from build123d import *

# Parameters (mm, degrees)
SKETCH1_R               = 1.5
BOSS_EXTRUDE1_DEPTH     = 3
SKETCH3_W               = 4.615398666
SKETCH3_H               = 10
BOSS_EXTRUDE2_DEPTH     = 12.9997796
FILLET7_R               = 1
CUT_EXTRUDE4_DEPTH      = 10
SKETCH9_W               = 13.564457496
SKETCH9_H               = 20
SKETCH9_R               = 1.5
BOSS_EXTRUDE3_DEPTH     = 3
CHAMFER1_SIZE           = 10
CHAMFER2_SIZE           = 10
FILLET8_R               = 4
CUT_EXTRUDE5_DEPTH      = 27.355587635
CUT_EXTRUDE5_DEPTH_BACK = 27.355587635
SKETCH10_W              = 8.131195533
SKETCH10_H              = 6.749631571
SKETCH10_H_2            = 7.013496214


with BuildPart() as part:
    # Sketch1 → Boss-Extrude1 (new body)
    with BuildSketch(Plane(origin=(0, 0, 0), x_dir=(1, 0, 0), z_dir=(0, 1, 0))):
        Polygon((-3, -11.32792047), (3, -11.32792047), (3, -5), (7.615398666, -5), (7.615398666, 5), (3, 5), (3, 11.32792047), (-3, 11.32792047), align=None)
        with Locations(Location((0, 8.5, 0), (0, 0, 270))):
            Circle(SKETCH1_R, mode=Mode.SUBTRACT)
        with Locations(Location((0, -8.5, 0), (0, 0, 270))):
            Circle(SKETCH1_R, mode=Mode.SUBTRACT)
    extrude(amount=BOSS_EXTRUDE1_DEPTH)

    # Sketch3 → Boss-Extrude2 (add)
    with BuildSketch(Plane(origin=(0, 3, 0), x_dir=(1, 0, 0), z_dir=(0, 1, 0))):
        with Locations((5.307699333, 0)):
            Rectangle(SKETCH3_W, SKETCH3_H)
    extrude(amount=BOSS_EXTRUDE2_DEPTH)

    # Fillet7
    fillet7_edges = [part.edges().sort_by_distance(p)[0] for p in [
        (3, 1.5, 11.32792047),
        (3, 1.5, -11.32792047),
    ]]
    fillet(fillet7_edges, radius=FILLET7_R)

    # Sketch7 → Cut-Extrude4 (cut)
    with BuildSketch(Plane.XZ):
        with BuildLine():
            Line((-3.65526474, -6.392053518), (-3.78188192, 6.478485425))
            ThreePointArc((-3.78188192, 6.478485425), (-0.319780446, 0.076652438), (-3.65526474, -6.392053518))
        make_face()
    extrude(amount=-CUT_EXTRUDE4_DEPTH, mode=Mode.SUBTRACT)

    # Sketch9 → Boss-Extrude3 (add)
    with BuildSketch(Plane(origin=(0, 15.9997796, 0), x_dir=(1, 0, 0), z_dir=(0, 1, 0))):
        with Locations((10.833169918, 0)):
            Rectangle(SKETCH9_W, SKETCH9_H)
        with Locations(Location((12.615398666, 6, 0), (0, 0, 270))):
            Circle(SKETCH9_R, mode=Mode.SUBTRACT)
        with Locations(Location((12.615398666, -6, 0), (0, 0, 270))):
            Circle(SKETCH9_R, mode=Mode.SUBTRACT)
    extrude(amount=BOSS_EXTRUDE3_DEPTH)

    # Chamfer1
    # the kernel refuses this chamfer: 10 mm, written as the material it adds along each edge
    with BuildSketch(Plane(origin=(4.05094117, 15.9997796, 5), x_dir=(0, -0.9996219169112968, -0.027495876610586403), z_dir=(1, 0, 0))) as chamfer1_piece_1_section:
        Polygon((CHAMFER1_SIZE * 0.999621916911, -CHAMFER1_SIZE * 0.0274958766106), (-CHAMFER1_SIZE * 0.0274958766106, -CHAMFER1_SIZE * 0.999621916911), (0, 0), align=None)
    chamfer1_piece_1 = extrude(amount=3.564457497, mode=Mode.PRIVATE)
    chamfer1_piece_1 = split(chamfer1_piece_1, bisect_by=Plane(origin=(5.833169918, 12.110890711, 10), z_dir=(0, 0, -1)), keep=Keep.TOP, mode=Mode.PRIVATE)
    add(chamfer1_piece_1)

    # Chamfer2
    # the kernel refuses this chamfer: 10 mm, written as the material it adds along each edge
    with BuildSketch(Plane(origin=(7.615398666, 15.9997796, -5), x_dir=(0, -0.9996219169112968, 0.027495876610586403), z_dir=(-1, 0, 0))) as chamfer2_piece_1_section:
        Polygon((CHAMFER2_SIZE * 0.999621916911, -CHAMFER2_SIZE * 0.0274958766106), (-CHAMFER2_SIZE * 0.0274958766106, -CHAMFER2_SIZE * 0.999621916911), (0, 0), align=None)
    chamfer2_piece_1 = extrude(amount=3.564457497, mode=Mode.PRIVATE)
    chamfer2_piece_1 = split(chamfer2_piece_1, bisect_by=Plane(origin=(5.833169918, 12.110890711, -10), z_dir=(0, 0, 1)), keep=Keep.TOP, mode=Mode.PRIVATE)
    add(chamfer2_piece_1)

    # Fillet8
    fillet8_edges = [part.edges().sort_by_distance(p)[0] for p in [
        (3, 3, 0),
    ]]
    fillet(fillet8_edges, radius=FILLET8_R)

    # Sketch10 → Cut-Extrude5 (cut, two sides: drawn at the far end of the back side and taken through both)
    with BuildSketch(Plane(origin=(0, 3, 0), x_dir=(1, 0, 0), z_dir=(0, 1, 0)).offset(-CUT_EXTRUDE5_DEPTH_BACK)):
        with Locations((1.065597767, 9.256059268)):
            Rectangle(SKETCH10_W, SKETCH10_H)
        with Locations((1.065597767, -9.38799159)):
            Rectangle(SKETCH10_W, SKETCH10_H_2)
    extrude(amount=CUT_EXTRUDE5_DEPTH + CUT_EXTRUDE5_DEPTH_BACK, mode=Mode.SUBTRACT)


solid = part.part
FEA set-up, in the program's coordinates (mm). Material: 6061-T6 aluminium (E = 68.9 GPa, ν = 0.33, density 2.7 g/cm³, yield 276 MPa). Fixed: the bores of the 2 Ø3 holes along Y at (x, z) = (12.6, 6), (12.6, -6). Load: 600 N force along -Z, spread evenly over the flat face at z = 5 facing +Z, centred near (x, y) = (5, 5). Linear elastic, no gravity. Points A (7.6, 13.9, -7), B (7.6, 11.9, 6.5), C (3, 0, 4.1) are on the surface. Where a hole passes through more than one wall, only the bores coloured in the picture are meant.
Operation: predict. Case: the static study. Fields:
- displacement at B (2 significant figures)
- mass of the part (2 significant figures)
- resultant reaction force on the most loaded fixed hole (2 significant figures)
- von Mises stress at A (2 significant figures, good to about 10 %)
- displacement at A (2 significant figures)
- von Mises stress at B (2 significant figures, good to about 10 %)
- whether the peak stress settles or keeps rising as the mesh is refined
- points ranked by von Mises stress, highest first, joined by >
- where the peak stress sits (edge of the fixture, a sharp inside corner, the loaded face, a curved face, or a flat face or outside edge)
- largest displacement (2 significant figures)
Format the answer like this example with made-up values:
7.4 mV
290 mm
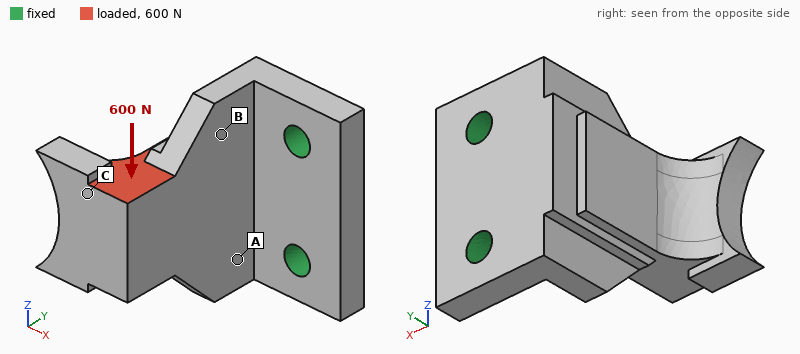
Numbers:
25 µm
5.0 g
690 N
65 MPa
21 µm
41 MPa
keeps rising
A > B > C
edge of the fixture
57 µm
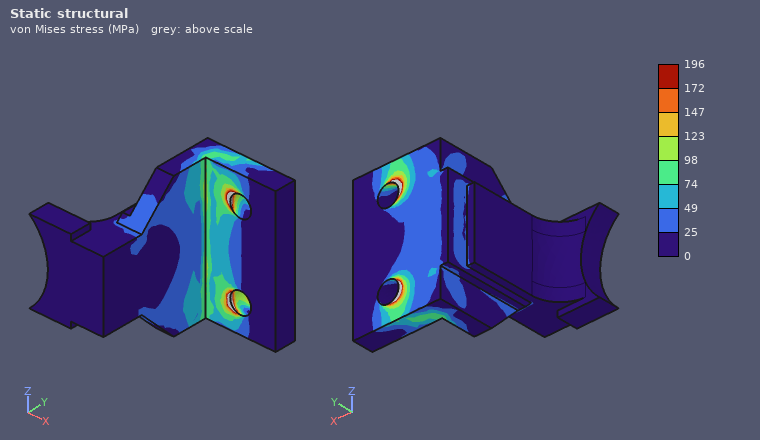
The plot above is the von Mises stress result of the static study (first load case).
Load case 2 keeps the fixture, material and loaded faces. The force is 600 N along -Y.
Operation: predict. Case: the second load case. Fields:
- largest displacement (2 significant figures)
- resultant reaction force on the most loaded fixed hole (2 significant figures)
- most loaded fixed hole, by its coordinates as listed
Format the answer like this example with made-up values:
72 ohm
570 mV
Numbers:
0.14 mm
510 N
(12.6, 6)
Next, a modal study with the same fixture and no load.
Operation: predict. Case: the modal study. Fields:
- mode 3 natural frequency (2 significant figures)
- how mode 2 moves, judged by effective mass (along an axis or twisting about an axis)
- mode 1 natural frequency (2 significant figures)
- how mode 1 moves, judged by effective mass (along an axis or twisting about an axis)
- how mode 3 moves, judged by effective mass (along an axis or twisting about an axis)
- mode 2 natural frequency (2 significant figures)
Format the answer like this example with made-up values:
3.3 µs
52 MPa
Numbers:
22 kHz
along Z
4800 Hz
along X
along Y
12 kHz
